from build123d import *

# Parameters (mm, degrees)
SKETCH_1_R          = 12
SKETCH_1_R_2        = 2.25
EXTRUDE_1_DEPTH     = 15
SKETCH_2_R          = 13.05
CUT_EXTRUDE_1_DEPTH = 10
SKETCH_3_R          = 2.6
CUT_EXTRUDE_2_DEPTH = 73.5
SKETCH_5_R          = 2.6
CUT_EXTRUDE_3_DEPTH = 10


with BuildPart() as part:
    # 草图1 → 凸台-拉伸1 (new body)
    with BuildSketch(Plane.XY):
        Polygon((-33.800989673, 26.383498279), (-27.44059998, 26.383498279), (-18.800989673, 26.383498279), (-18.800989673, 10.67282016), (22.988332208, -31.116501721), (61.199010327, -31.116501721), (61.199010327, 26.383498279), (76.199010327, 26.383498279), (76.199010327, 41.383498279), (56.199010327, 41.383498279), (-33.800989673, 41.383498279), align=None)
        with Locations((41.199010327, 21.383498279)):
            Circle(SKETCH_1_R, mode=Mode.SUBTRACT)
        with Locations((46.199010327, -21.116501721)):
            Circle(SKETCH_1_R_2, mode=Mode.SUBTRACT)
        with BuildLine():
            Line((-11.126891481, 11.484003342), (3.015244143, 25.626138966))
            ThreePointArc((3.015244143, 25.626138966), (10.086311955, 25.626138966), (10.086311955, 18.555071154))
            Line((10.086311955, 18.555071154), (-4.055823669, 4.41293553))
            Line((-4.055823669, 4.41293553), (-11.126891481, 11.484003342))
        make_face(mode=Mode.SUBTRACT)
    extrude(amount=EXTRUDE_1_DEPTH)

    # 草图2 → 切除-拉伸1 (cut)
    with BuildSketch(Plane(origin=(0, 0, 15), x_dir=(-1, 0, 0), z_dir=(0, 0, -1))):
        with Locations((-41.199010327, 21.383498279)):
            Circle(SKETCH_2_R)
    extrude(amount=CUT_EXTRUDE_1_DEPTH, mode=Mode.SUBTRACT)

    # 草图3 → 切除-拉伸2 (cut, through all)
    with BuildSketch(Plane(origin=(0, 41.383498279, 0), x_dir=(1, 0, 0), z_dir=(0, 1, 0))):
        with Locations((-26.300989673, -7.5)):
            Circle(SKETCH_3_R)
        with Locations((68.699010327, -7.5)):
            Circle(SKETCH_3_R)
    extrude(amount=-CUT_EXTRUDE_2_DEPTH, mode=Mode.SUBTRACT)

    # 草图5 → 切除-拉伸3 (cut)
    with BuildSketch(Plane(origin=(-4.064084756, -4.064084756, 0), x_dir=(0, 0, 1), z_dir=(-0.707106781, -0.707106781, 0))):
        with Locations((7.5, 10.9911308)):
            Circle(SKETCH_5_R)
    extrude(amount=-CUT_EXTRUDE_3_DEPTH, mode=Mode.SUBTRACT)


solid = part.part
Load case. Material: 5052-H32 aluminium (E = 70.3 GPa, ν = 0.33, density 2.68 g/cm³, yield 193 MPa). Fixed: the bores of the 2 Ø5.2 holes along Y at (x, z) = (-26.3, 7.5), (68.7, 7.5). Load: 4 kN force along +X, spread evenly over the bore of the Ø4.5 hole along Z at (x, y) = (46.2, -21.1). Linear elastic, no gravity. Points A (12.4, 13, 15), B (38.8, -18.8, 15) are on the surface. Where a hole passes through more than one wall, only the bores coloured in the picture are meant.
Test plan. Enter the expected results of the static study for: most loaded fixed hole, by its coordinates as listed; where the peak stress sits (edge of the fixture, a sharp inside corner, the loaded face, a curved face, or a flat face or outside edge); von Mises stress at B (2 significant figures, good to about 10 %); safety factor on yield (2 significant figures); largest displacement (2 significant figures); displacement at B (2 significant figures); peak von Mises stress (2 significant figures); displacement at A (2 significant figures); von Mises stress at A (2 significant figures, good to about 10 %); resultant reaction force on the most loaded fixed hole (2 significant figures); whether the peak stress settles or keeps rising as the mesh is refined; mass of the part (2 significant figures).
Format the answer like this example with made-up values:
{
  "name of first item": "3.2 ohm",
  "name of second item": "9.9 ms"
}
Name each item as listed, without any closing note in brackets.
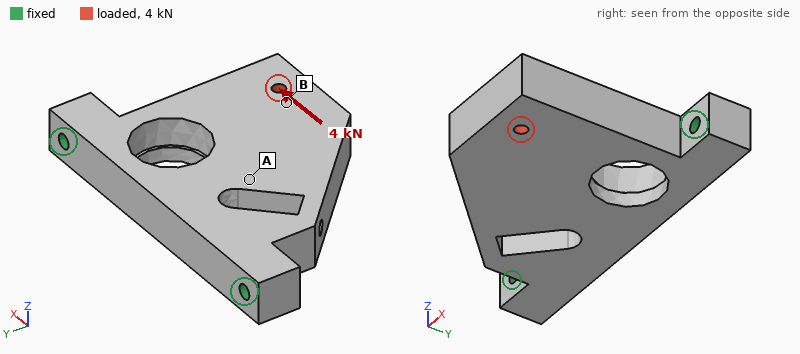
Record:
{
  "most loaded fixed hole, by its coordinates as listed": "(-26.3, 7.5)",
  "where the peak stress sits": "a curved face",
  "von Mises stress at B": "15 MPa",
  "safety factor on yield": "1.9",
  "largest displacement": "45 µm",
  "displacement at B": "35 µm",
  "peak von Mises stress": "100 MPa",
  "displacement at A": "18 µm",
  "von Mises stress at A": "5.0 MPa",
  "resultant reaction force on the most loaded fixed hole": "3.6 kN",
  "whether the peak stress settles or keeps rising as the mesh is refined": "settles",
  "mass of the part": "180 g"
}
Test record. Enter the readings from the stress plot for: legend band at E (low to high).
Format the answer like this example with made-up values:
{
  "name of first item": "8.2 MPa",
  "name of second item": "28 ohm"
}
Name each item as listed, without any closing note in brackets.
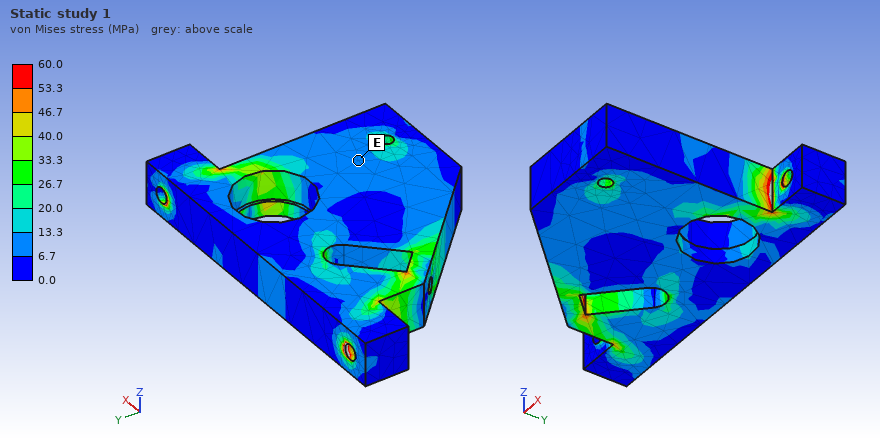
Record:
{
  "legend band at E": "6.7 to 13.3 MPa"
}
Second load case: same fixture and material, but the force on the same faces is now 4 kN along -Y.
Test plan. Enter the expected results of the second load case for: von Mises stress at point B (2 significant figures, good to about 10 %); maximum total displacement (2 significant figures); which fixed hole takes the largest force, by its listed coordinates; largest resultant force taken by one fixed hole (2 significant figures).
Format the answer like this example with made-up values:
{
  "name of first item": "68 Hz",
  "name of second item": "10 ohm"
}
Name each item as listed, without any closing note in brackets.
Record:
{
  "von Mises stress at point B": "6.2 MPa",
  "maximum total displacement": "22 µm",
  "which fixed hole takes the largest force, by its listed coordinates": "(68.7, 7.5)",
  "largest resultant force taken by one fixed hole": "3.2 kN"
}
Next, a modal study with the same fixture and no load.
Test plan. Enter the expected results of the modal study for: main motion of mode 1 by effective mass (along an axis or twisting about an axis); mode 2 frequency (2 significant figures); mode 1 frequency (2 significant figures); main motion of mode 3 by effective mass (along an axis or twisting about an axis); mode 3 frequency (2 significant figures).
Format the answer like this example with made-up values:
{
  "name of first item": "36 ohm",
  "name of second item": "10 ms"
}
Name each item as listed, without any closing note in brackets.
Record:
{
  "main motion of mode 1 by effective mass": "along Z",
  "mode 2 frequency": "5200 Hz",
  "mode 1 frequency": "1500 Hz",
  "main motion of mode 3 by effective mass": "along X",
  "mode 3 frequency": "6200 Hz"
}
